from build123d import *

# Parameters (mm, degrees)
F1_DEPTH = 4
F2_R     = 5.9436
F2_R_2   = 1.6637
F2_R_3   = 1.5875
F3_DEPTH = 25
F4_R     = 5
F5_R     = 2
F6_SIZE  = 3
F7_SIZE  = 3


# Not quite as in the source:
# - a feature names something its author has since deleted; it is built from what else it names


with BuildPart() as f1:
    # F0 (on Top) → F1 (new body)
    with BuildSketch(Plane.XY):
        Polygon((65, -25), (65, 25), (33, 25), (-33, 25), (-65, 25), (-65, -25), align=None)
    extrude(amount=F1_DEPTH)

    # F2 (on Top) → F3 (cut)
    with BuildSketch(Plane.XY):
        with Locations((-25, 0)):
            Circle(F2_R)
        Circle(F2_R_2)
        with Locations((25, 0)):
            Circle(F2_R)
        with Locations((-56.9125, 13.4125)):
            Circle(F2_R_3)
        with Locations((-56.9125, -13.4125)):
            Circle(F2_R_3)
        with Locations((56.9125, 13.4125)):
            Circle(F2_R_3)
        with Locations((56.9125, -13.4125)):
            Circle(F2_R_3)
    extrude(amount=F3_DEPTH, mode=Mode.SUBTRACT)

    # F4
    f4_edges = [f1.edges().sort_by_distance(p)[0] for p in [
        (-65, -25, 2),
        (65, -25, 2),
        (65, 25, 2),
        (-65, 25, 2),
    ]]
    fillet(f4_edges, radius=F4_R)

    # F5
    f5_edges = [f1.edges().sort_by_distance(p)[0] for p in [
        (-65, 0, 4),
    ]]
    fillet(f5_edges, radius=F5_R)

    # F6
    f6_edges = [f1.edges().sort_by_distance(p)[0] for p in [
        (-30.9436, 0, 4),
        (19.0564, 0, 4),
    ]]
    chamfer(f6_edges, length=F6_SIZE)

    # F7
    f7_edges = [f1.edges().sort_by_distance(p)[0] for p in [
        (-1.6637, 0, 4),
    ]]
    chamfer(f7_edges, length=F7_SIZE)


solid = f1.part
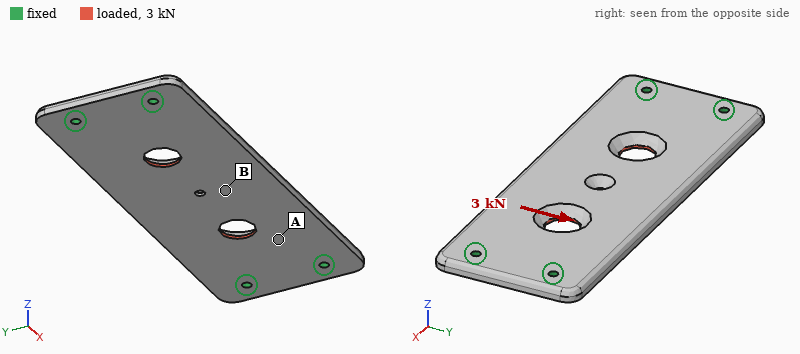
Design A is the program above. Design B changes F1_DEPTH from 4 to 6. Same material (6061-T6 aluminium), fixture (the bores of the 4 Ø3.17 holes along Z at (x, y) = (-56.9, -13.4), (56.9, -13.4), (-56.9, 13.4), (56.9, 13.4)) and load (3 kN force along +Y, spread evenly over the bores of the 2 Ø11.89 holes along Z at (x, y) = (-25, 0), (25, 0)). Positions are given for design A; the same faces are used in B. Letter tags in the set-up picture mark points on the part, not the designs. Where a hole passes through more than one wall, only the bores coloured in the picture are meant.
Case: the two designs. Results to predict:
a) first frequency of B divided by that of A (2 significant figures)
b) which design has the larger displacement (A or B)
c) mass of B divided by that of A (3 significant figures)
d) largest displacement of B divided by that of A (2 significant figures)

1.4
A
1.52
0.41
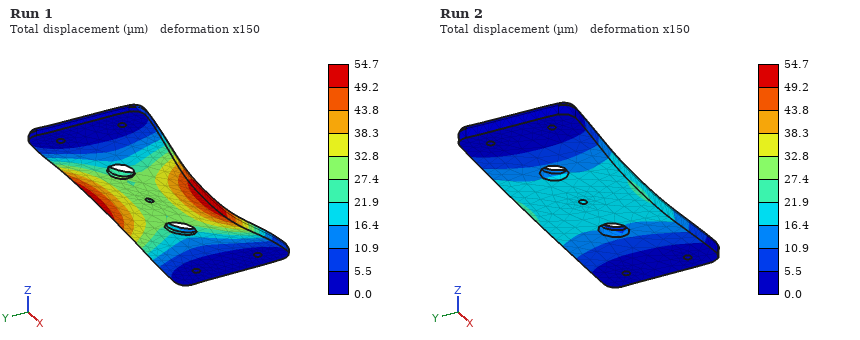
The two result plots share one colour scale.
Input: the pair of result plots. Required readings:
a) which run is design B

Run 2
